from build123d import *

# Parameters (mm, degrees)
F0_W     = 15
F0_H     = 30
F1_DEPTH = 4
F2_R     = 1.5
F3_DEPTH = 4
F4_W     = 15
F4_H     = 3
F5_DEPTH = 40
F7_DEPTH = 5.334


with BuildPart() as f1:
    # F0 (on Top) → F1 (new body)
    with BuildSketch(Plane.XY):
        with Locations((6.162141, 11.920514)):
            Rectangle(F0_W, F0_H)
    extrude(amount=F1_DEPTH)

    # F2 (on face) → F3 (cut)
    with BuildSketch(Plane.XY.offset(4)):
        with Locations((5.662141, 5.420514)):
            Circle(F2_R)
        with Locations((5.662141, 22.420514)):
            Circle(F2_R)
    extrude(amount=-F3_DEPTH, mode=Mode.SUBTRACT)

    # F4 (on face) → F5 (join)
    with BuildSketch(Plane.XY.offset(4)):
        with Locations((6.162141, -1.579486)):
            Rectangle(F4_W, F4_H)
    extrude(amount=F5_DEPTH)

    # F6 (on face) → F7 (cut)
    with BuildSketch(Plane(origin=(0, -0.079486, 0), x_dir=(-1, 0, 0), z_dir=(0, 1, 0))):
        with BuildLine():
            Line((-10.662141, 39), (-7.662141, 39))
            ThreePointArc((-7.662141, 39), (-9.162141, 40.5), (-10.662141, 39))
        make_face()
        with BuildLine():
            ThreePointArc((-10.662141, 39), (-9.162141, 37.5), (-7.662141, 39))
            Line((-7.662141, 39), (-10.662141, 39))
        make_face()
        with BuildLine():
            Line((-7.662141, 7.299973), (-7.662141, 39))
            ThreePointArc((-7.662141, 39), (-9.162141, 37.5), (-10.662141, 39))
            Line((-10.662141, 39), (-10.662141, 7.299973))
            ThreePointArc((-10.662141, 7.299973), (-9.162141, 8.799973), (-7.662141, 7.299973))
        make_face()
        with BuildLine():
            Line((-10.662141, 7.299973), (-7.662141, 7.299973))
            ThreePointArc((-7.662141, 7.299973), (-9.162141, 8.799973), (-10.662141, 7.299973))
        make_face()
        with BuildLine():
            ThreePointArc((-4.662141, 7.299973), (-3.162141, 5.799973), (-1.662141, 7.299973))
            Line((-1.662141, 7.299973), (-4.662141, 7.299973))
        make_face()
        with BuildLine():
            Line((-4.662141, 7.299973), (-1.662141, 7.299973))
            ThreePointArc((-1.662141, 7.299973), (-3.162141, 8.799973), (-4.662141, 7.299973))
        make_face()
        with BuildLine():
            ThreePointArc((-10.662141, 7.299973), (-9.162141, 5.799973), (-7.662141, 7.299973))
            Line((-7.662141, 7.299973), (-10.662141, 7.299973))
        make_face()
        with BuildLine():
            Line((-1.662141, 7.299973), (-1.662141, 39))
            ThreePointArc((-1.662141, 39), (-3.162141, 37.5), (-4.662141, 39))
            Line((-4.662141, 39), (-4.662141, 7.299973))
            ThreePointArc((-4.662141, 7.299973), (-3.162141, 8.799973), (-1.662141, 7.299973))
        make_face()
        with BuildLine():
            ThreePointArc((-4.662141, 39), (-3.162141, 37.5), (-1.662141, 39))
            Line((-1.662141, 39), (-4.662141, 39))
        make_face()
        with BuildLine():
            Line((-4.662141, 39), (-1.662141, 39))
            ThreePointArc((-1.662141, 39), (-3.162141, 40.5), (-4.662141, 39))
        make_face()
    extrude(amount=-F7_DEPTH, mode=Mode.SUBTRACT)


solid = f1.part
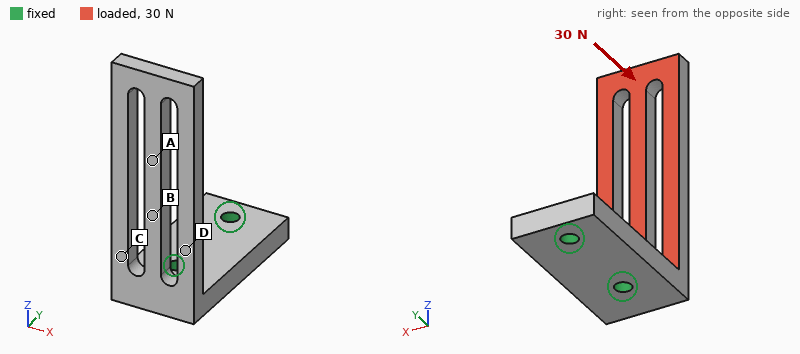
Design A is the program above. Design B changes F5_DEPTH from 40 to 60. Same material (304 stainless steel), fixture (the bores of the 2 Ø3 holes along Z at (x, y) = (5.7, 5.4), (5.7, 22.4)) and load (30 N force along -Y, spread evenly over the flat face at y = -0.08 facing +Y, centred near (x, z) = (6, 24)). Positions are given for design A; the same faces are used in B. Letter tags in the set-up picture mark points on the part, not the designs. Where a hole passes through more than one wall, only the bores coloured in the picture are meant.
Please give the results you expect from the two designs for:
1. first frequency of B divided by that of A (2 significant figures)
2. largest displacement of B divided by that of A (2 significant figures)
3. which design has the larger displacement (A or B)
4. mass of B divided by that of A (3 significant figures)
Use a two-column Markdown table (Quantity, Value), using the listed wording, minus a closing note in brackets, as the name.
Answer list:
| Quantity | Value |
|---|---|
| first frequency of B divided by that of A | 0.40 |
| largest displacement of B divided by that of A | 3.4 |
| which design has the larger displacement | B |
| mass of B divided by that of A | 1.31 |
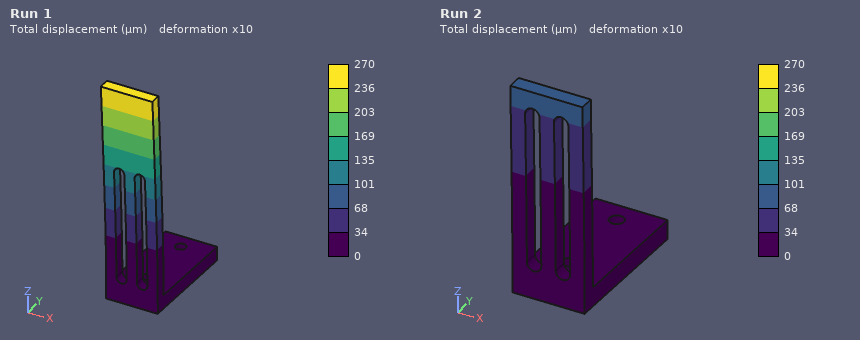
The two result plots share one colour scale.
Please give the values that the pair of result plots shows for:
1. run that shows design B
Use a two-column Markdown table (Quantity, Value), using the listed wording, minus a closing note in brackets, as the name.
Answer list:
| Quantity | Value |
|---|---|
| run that shows design B | Run 1 |
